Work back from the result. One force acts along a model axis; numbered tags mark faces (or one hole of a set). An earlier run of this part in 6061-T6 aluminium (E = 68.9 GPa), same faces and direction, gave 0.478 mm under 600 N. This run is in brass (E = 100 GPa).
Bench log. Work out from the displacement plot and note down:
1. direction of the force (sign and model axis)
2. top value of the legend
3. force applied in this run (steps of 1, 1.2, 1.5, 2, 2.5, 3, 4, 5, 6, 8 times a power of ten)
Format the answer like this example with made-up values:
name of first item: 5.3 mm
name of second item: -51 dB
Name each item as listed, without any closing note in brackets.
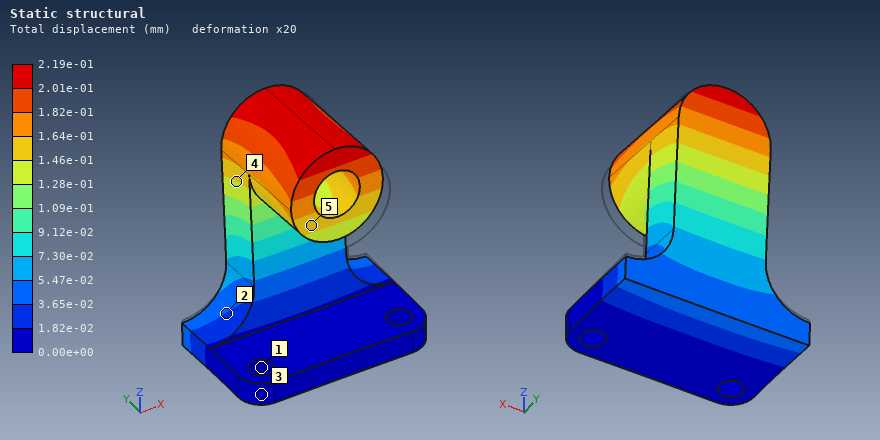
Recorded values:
direction of the force: +Y
top value of the legend: 2.19e-01 mm
force applied in this run: 400 N
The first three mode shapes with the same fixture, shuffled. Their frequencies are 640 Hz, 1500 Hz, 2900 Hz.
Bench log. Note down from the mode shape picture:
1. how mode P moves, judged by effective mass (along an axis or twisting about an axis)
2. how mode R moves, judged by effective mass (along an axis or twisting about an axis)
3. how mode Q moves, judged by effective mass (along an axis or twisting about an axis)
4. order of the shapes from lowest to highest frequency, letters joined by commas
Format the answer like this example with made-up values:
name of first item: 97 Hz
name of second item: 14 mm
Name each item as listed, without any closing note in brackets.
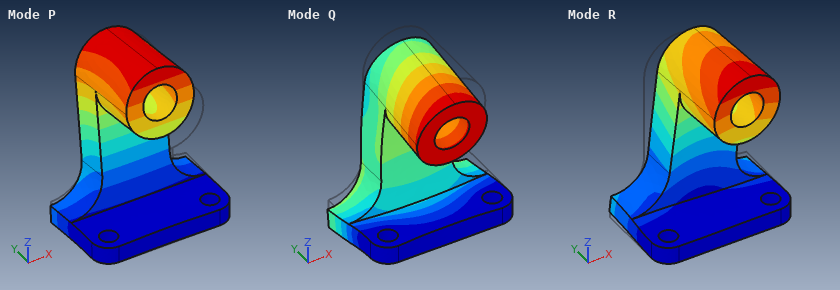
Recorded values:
how mode P moves, judged by effective mass: along Y
how mode R moves, judged by effective mass: along X
how mode Q moves, judged by effective mass: along Z
order of the shapes from lowest to highest frequency, letters joined by commas: P, R, Q
